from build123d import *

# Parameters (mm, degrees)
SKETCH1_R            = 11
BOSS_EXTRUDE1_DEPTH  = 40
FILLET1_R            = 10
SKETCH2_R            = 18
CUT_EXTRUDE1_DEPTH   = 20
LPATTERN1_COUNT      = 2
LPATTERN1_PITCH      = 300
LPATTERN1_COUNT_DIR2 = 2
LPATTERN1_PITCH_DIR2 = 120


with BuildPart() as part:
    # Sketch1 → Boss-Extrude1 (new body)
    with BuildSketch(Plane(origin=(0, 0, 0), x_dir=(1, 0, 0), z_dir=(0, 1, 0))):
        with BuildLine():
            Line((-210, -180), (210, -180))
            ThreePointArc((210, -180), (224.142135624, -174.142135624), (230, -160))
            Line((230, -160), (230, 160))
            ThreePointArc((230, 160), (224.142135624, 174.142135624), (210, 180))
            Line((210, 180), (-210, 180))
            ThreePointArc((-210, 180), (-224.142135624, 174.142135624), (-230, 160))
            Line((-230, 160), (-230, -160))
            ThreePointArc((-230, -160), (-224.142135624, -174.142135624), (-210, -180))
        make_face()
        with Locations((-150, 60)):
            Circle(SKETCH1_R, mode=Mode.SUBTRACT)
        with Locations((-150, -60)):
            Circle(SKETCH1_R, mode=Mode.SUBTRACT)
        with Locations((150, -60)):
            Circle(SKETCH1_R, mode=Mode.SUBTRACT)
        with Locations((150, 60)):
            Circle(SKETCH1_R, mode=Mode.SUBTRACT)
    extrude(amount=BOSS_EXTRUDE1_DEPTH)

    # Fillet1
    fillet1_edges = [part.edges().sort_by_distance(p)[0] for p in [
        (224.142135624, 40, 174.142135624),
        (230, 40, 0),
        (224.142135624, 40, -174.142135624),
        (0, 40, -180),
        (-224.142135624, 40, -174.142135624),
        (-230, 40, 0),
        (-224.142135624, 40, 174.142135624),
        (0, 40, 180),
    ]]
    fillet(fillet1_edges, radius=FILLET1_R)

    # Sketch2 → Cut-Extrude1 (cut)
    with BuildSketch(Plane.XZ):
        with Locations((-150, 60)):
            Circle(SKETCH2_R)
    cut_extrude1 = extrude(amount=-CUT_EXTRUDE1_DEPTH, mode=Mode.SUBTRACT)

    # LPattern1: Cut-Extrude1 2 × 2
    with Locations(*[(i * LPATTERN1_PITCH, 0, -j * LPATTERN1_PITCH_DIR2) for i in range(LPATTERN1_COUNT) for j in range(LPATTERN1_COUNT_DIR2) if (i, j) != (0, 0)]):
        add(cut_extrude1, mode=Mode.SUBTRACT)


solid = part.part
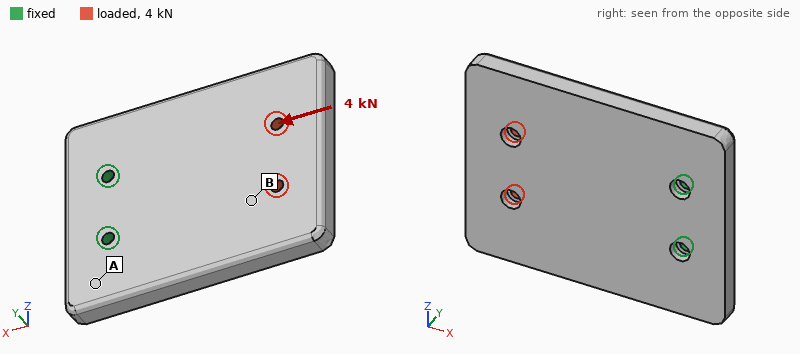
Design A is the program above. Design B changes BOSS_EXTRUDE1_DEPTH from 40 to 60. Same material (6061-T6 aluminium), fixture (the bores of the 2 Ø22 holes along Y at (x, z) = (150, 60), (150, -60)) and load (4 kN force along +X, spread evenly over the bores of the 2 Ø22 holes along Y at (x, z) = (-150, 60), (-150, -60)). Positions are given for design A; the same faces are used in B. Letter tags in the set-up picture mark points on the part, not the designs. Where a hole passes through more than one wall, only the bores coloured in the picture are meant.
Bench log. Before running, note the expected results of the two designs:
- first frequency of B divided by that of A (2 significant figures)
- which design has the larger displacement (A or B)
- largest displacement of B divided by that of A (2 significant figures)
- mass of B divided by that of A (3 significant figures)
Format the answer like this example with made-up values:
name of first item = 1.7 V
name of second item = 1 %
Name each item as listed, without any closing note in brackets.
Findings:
first frequency of B divided by that of A = 1.6
which design has the larger displacement = A
largest displacement of B divided by that of A = 0.31
mass of B divided by that of A = 1.51
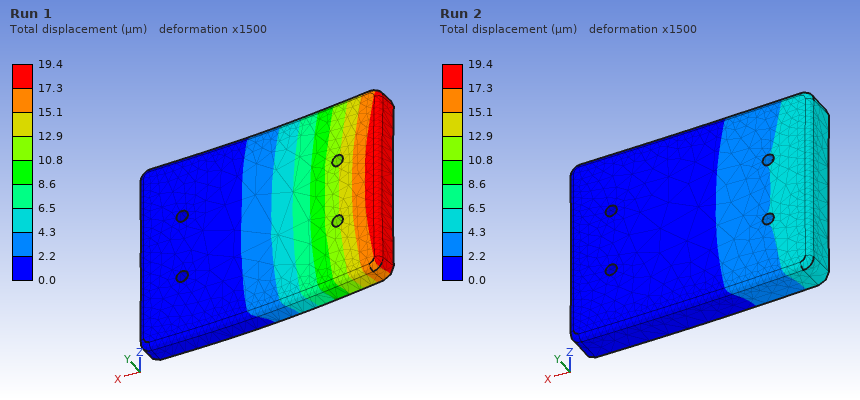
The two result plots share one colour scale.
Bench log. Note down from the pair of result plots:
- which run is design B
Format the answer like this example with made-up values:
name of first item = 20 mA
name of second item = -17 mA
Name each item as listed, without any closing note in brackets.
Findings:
which run is design B = Run 2
